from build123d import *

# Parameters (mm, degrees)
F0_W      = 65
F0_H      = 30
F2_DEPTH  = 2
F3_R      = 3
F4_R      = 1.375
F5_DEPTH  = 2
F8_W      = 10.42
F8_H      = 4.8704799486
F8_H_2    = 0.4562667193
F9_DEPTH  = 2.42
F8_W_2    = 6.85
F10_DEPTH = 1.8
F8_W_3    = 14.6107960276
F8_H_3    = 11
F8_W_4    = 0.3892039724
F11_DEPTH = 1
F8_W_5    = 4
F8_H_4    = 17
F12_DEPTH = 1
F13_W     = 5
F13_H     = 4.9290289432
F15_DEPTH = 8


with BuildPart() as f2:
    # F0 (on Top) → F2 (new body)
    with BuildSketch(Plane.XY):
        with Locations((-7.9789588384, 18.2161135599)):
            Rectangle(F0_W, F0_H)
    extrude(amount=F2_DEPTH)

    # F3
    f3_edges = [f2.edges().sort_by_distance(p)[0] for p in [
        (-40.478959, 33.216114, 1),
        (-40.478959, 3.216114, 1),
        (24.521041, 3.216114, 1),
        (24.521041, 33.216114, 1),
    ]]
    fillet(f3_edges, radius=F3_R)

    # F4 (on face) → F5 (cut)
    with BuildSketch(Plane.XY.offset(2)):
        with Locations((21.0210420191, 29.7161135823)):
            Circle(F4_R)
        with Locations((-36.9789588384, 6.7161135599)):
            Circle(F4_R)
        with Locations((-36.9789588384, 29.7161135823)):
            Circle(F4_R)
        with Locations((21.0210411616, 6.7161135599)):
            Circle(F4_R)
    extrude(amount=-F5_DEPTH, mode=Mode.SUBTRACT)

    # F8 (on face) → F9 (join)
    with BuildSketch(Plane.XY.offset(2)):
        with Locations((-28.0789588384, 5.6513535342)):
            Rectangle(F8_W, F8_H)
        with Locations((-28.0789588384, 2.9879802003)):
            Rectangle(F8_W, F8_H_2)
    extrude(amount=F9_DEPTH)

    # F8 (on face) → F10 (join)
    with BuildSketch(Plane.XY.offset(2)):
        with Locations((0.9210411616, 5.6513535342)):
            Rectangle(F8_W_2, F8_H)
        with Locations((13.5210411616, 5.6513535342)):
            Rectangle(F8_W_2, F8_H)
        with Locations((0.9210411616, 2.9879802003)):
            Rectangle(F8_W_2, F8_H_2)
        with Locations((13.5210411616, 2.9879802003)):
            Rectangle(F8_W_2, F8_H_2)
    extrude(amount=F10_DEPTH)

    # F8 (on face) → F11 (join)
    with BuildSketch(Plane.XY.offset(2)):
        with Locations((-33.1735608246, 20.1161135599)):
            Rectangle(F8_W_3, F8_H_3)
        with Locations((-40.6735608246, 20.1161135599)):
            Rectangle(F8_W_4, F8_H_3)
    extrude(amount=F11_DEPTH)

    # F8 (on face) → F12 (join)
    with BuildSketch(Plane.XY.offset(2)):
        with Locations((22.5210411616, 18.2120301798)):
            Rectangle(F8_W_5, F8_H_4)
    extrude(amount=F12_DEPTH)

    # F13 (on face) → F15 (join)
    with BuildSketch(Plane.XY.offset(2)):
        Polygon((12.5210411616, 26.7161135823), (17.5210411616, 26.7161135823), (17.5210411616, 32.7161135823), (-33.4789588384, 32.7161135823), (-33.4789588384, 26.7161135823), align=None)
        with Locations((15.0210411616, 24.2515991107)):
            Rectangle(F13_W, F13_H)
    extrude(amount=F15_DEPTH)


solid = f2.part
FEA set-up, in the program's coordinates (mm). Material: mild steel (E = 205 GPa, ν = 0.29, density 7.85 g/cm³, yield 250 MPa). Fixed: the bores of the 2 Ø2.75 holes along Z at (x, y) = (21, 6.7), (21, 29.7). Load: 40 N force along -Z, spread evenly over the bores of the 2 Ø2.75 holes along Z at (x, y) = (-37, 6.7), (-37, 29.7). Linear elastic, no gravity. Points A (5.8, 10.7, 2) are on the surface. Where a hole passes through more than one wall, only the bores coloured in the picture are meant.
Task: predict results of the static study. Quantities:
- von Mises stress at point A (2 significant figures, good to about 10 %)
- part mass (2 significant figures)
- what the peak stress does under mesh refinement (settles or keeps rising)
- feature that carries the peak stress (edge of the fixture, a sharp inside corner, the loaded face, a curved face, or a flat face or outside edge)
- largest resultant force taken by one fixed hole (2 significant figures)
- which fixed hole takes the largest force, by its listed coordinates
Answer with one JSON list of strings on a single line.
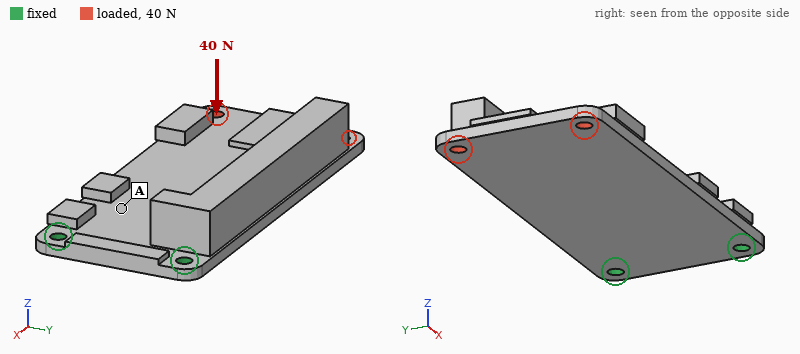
["21 MPa", "55 g", "keeps rising", "edge of the fixture", "29 N", "(21, 6.7)"]
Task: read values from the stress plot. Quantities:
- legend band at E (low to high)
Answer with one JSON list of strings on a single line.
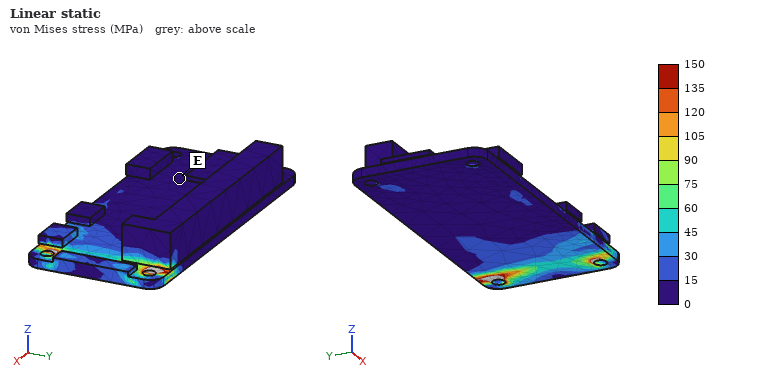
["0 to 15 MPa"]
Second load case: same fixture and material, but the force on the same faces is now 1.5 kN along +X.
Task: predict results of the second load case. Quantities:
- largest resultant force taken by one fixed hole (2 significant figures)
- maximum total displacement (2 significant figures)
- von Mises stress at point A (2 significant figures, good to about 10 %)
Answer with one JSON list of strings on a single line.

["760 N", "32 µm", "22 MPa"]
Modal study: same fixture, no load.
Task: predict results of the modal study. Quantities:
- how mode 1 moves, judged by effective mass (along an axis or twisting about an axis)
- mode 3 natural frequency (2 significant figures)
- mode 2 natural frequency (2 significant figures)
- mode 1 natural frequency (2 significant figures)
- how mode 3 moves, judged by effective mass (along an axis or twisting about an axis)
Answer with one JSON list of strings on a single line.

["along Z", "4400 Hz", "2500 Hz", "530 Hz", "along Y"]
